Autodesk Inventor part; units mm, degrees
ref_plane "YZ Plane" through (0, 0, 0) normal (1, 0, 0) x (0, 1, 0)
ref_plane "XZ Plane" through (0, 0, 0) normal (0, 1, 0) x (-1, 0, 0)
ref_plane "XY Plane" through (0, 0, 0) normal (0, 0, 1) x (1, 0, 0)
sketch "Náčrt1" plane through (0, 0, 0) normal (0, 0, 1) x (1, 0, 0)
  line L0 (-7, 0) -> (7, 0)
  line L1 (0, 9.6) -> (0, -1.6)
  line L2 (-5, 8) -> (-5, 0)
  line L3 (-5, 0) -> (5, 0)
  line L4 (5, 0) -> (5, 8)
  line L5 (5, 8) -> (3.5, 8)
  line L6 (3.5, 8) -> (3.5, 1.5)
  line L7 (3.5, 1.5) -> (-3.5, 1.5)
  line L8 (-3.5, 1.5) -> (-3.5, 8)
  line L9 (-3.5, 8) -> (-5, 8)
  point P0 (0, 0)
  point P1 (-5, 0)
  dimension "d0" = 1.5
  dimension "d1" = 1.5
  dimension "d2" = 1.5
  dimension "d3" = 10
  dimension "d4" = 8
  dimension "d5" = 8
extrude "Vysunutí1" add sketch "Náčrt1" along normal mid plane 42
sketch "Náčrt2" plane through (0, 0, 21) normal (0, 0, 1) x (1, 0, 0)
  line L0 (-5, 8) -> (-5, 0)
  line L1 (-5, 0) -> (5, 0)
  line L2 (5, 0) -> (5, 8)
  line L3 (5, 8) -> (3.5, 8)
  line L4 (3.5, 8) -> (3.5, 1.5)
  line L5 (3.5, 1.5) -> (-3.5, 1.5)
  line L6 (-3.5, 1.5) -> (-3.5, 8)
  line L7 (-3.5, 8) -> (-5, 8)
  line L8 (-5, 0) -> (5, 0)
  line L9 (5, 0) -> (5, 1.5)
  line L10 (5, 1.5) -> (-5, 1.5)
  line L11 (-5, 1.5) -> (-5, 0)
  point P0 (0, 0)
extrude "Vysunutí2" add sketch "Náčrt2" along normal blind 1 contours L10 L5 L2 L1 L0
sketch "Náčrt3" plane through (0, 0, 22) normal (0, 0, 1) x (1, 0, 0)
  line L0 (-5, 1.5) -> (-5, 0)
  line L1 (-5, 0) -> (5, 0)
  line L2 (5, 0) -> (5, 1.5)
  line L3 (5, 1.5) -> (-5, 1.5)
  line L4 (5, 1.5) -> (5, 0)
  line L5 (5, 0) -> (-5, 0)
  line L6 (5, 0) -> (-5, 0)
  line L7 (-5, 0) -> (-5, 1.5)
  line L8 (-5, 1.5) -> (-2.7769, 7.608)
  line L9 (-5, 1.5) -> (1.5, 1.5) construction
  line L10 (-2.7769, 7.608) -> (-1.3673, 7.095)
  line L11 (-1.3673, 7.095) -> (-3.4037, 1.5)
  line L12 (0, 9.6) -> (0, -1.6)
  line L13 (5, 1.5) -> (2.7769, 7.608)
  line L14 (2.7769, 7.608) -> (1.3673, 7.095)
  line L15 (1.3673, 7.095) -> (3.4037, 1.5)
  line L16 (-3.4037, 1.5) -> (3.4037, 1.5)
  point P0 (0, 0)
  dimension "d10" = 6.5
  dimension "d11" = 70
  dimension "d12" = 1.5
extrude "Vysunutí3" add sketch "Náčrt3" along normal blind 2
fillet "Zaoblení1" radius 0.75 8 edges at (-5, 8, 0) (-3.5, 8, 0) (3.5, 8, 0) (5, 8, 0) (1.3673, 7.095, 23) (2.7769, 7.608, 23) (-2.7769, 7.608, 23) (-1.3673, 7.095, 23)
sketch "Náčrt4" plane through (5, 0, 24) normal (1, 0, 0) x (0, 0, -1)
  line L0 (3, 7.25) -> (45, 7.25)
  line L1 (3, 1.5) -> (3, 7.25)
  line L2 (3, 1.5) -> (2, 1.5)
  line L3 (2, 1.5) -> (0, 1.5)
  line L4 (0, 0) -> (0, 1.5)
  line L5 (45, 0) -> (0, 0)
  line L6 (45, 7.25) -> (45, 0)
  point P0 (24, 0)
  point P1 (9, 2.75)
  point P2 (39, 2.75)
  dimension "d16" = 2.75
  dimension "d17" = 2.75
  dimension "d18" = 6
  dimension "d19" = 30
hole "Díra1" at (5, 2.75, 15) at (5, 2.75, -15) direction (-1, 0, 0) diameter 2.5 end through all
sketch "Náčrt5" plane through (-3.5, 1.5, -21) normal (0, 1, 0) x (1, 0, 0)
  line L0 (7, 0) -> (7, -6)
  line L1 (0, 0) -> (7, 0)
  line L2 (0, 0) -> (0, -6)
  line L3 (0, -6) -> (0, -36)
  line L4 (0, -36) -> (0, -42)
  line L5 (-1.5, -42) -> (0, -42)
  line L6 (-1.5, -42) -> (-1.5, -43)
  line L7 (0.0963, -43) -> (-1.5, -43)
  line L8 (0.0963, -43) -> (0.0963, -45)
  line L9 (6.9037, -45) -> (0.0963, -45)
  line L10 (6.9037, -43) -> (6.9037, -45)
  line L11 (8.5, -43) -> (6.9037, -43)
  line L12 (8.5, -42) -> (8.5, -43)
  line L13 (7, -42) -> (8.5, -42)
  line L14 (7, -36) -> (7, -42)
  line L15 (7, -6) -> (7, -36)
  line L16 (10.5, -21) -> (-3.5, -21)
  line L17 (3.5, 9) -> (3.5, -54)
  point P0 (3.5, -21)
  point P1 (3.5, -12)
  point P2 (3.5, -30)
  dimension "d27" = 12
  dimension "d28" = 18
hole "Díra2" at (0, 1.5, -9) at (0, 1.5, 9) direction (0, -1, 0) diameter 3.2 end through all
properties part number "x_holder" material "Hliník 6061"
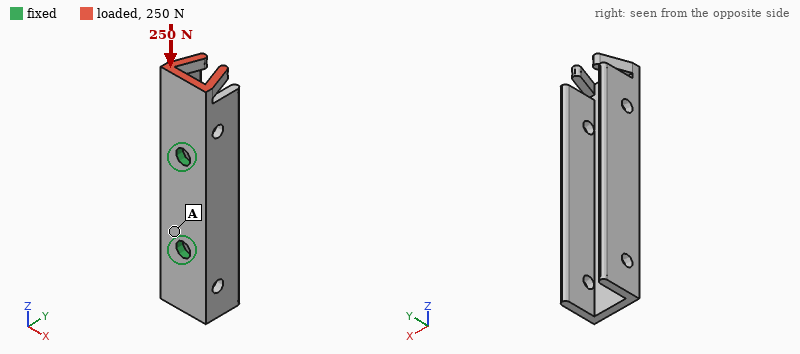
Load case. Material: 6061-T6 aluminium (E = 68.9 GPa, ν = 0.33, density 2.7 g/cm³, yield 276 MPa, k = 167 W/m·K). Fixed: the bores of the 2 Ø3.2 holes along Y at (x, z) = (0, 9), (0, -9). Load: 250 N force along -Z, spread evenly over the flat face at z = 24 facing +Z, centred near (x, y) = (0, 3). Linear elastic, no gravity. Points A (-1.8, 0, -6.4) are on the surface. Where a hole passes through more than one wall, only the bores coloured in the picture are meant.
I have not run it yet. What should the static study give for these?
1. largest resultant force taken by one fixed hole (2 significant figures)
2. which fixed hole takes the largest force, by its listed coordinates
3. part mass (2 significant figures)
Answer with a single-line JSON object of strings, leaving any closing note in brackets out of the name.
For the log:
{"largest resultant force taken by one fixed hole": "190 N", "which fixed hole takes the largest force, by its listed coordinates": "(0, 9)", "part mass": "3.9 g"}
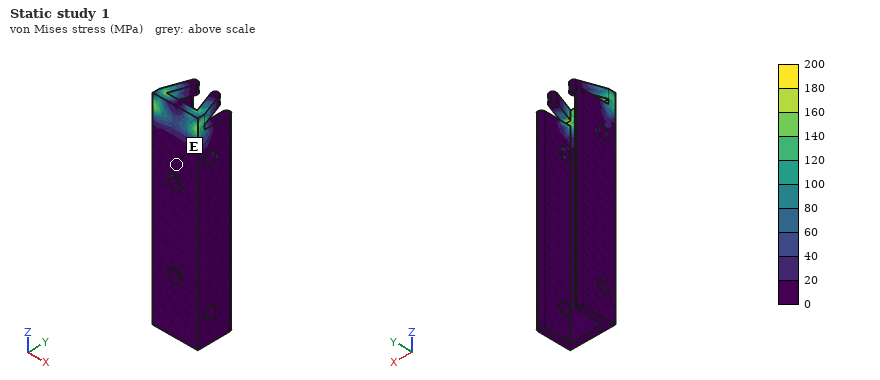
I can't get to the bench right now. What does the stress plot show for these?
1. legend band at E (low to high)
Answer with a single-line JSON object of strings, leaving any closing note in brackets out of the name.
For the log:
{"legend band at E": "0 to 20 MPa"}
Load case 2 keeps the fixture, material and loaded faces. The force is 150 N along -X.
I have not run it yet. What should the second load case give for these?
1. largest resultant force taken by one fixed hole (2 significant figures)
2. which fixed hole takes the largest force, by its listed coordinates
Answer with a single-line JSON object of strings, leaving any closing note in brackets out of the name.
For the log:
{"largest resultant force taken by one fixed hole": "220 N", "which fixed hole takes the largest force, by its listed coordinates": "(0, 9)"}
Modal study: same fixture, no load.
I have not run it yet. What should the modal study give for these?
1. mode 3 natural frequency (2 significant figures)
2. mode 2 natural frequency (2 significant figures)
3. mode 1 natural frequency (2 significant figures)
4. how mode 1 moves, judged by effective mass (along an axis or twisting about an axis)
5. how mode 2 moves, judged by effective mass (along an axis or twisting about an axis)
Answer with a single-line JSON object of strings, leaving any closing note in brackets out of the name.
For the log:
{"mode 3 natural frequency": "13 kHz", "mode 2 natural frequency": "11 kHz", "mode 1 natural frequency": "10 kHz", "how mode 1 moves, judged by effective mass": "along X", "how mode 2 moves, judged by effective mass": "along X"}
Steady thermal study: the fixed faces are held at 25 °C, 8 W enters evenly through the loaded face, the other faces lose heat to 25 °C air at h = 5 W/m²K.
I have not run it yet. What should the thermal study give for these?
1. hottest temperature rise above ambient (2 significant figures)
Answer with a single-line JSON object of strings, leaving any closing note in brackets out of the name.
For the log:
{"hottest temperature rise above ambient": "47 K"}
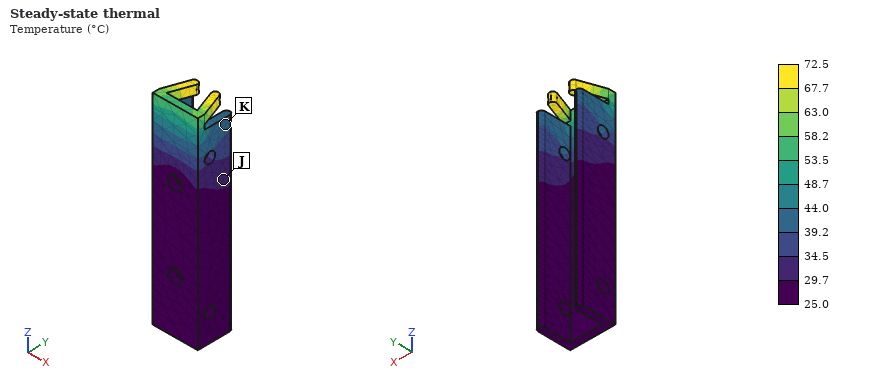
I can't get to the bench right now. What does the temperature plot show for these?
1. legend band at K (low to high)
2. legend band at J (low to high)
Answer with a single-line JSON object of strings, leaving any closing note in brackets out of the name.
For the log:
{"legend band at K": "39.2 to 44.0 °C", "legend band at J": "29.7 to 34.5 °C"}
